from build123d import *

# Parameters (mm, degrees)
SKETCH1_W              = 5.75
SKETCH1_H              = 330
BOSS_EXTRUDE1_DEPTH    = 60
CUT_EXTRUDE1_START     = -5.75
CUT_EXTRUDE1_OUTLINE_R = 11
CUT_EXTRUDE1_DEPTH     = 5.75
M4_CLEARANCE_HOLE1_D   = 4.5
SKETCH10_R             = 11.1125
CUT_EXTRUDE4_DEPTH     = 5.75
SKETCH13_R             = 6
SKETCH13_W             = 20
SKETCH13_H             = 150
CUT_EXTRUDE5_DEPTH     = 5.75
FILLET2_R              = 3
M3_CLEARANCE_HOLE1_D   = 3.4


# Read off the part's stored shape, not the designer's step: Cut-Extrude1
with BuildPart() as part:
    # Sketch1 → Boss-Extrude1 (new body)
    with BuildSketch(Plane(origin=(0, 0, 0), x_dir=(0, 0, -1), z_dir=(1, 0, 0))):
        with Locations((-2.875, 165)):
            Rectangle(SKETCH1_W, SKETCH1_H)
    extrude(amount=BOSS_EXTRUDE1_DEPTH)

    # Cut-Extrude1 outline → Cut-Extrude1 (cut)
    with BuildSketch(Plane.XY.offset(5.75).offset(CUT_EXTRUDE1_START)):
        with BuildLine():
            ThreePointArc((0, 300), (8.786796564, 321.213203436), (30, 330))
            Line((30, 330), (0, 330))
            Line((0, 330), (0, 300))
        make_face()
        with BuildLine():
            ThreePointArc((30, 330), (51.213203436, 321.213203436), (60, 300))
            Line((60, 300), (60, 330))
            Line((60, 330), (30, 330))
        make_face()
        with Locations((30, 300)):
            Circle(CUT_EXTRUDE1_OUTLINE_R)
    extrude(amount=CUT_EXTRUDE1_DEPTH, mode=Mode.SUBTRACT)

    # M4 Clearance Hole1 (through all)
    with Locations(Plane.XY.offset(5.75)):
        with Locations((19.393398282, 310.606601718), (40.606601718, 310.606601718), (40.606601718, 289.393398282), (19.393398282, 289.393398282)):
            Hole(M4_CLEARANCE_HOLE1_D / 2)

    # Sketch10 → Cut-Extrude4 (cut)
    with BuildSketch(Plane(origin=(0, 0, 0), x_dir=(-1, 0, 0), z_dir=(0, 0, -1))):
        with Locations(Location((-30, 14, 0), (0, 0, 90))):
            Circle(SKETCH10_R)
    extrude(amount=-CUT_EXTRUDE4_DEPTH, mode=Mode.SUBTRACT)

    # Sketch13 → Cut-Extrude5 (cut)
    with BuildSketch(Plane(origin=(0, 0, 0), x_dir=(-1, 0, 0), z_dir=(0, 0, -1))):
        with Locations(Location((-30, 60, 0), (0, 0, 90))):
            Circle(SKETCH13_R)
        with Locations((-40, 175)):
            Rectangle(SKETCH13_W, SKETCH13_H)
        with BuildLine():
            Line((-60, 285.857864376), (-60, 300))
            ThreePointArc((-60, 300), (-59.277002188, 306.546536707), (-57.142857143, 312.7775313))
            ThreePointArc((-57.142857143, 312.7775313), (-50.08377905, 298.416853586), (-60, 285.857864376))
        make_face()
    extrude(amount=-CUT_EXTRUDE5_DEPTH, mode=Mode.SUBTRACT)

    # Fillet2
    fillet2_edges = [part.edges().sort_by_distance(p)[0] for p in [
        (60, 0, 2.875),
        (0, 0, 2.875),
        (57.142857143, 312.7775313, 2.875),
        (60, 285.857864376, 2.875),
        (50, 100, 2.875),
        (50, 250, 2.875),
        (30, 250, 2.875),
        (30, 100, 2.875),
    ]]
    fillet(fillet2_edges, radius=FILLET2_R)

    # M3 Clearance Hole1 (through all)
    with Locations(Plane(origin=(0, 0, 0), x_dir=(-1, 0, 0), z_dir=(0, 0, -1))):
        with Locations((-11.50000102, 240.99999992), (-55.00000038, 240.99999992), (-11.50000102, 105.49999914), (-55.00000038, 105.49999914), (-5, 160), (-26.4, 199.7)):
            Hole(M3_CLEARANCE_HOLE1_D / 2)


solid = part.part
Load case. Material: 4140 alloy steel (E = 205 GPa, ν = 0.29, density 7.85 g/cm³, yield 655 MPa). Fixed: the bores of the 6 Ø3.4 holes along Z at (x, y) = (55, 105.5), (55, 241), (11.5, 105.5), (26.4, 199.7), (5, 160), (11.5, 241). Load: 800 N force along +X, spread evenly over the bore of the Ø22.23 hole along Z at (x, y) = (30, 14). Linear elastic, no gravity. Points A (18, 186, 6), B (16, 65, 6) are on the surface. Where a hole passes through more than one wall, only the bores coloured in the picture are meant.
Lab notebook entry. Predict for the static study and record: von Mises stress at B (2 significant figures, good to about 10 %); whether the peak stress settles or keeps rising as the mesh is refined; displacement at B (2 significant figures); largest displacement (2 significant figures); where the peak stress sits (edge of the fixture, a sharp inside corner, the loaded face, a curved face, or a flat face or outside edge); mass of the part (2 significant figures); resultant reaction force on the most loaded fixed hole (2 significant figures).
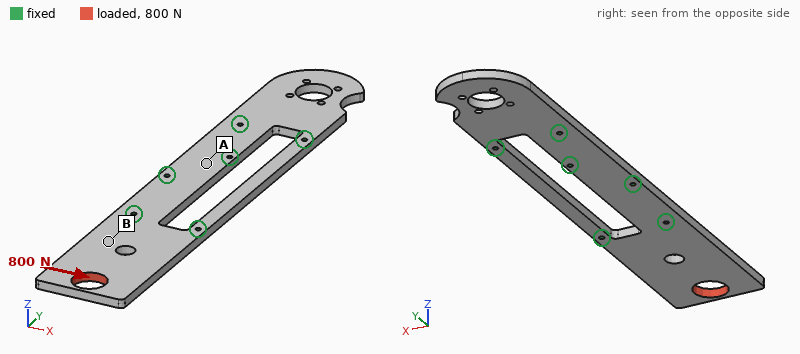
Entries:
8.6 MPa
keeps rising
5.2 µm
20 µm
edge of the fixture
690 g
1.6 kN
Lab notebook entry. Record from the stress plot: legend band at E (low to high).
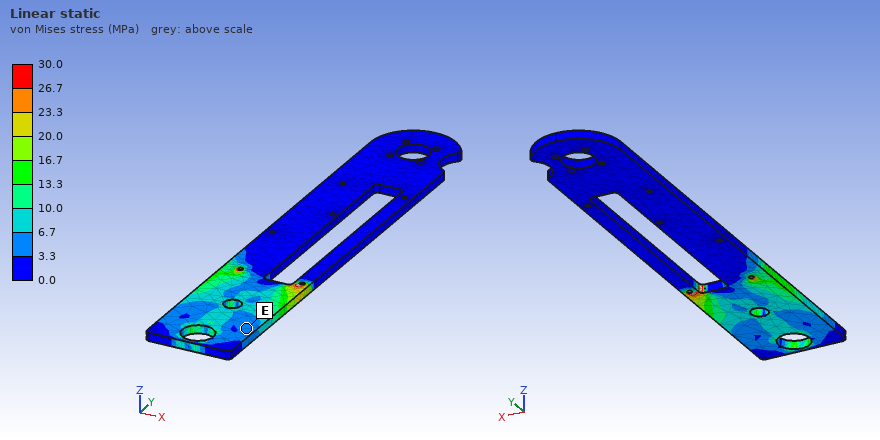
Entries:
3.3 to 6.7 MPa
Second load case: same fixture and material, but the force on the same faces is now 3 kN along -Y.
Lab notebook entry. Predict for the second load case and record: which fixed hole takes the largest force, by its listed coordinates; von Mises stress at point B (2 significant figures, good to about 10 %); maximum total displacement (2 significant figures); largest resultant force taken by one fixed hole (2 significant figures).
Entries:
(11.5, 105.5)
10 MPa
10 µm
1.5 kN
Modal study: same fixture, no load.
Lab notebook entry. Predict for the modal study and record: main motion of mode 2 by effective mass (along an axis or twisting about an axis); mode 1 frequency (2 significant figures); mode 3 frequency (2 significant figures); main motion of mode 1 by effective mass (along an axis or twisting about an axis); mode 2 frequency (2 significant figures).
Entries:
along Z
410 Hz
1500 Hz
along Z
640 Hz
